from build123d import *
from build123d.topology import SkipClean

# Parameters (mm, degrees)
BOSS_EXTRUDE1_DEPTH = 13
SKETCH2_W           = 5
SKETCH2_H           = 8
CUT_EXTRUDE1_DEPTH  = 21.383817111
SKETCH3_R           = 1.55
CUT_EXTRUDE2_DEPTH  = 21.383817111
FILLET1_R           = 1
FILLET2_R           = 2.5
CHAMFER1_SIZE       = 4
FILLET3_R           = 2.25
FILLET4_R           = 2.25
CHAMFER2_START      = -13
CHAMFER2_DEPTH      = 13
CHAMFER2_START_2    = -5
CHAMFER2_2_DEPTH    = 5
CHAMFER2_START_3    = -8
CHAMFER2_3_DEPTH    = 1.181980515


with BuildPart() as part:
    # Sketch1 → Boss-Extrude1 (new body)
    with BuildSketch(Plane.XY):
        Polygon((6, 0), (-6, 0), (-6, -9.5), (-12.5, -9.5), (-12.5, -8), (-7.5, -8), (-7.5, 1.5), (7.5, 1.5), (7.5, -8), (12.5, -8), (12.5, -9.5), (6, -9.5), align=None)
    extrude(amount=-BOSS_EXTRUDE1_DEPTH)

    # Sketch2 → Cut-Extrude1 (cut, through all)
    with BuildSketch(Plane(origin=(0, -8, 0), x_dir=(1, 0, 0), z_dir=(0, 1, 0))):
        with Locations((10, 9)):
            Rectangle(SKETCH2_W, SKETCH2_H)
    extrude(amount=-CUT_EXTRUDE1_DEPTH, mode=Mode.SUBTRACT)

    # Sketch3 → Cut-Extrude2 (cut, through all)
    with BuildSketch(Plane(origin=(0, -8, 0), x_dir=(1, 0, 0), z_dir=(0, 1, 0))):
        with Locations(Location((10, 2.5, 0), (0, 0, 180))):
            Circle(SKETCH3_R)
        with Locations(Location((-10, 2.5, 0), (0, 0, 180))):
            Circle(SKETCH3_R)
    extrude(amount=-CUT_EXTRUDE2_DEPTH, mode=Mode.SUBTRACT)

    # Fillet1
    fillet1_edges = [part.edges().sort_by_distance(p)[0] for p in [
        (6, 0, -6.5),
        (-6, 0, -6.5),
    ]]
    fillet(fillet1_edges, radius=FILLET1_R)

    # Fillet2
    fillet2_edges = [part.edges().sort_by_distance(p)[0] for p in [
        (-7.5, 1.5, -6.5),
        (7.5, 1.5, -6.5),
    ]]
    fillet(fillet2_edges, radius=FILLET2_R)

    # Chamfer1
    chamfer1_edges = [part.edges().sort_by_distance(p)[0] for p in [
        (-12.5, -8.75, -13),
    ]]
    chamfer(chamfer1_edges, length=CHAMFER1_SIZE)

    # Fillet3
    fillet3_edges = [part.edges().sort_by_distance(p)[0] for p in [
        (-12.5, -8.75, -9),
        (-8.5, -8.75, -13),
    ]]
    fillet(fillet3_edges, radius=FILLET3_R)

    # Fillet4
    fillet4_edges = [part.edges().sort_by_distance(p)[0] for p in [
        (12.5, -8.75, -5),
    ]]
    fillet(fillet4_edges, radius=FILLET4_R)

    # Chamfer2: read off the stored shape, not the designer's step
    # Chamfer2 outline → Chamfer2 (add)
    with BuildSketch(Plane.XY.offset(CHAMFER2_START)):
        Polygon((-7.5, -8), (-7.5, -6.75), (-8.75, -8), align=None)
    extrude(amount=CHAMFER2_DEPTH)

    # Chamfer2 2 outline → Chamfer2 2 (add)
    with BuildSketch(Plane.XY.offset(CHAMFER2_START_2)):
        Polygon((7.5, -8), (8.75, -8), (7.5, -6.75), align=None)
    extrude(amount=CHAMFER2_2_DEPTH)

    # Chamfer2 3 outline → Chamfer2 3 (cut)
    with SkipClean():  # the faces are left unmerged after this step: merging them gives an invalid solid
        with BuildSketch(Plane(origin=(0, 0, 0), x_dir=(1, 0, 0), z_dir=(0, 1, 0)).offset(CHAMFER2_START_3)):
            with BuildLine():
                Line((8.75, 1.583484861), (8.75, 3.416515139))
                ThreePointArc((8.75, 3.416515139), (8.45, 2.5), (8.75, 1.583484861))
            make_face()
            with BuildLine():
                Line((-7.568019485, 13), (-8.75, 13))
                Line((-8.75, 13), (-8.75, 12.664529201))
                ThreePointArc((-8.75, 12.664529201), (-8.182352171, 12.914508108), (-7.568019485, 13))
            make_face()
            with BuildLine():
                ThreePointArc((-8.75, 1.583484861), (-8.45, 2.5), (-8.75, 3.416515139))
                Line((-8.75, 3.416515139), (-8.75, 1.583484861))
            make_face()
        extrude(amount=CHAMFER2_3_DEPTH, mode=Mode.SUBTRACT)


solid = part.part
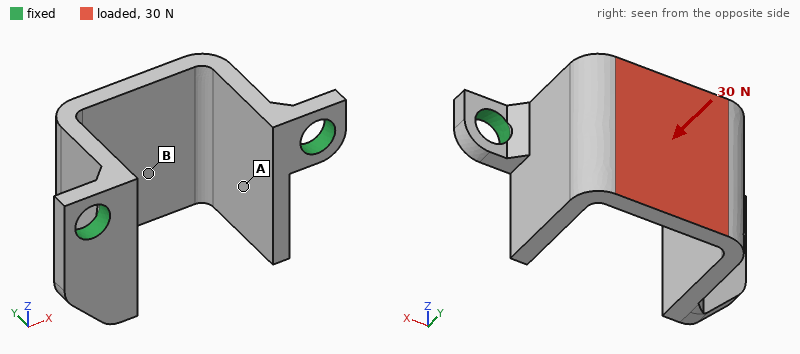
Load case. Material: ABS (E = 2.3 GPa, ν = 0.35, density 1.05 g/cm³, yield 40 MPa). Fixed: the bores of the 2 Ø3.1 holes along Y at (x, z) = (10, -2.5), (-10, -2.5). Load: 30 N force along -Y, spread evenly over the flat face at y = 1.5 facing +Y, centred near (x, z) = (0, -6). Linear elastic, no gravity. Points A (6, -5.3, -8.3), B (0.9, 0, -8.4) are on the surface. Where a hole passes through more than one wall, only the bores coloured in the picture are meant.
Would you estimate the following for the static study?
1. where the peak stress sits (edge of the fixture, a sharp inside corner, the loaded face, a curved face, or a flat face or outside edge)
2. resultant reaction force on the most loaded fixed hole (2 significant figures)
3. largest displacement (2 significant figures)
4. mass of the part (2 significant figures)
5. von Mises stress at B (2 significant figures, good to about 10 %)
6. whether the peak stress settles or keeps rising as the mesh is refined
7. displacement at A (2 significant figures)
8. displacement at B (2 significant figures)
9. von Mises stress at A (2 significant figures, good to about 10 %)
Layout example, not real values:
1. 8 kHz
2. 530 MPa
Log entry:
1. edge of the fixture
2. 16 N
3. 0.19 mm
4. 0.78 g
5. 4.8 MPa
6. keeps rising
7. 0.069 mm
8. 0.13 mm
9. 2.0 MPa
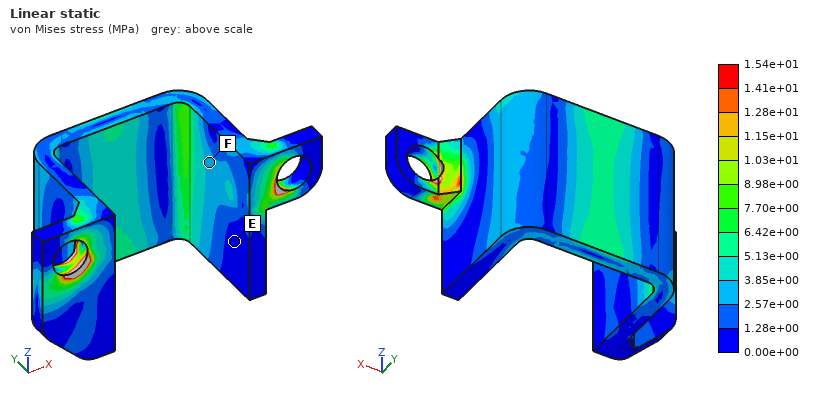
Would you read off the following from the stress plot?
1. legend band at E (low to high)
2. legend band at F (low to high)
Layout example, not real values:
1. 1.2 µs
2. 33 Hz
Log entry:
1. 0.00e+00 to 1.28e+00 MPa
2. 2.57e+00 to 3.85e+00 MPa
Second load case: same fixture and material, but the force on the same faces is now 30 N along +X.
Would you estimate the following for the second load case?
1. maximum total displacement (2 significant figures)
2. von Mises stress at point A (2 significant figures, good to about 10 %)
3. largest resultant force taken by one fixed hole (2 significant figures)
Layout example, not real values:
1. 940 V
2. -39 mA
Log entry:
1. 0.23 mm
2. 2.1 MPa
3. 21 N
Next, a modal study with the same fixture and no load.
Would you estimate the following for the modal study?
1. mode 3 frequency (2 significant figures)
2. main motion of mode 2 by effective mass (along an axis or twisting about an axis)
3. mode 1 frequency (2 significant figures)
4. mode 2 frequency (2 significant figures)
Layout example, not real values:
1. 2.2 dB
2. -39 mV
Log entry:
1. 3800 Hz
2. along X
3. 2400 Hz
4. 2800 Hz
